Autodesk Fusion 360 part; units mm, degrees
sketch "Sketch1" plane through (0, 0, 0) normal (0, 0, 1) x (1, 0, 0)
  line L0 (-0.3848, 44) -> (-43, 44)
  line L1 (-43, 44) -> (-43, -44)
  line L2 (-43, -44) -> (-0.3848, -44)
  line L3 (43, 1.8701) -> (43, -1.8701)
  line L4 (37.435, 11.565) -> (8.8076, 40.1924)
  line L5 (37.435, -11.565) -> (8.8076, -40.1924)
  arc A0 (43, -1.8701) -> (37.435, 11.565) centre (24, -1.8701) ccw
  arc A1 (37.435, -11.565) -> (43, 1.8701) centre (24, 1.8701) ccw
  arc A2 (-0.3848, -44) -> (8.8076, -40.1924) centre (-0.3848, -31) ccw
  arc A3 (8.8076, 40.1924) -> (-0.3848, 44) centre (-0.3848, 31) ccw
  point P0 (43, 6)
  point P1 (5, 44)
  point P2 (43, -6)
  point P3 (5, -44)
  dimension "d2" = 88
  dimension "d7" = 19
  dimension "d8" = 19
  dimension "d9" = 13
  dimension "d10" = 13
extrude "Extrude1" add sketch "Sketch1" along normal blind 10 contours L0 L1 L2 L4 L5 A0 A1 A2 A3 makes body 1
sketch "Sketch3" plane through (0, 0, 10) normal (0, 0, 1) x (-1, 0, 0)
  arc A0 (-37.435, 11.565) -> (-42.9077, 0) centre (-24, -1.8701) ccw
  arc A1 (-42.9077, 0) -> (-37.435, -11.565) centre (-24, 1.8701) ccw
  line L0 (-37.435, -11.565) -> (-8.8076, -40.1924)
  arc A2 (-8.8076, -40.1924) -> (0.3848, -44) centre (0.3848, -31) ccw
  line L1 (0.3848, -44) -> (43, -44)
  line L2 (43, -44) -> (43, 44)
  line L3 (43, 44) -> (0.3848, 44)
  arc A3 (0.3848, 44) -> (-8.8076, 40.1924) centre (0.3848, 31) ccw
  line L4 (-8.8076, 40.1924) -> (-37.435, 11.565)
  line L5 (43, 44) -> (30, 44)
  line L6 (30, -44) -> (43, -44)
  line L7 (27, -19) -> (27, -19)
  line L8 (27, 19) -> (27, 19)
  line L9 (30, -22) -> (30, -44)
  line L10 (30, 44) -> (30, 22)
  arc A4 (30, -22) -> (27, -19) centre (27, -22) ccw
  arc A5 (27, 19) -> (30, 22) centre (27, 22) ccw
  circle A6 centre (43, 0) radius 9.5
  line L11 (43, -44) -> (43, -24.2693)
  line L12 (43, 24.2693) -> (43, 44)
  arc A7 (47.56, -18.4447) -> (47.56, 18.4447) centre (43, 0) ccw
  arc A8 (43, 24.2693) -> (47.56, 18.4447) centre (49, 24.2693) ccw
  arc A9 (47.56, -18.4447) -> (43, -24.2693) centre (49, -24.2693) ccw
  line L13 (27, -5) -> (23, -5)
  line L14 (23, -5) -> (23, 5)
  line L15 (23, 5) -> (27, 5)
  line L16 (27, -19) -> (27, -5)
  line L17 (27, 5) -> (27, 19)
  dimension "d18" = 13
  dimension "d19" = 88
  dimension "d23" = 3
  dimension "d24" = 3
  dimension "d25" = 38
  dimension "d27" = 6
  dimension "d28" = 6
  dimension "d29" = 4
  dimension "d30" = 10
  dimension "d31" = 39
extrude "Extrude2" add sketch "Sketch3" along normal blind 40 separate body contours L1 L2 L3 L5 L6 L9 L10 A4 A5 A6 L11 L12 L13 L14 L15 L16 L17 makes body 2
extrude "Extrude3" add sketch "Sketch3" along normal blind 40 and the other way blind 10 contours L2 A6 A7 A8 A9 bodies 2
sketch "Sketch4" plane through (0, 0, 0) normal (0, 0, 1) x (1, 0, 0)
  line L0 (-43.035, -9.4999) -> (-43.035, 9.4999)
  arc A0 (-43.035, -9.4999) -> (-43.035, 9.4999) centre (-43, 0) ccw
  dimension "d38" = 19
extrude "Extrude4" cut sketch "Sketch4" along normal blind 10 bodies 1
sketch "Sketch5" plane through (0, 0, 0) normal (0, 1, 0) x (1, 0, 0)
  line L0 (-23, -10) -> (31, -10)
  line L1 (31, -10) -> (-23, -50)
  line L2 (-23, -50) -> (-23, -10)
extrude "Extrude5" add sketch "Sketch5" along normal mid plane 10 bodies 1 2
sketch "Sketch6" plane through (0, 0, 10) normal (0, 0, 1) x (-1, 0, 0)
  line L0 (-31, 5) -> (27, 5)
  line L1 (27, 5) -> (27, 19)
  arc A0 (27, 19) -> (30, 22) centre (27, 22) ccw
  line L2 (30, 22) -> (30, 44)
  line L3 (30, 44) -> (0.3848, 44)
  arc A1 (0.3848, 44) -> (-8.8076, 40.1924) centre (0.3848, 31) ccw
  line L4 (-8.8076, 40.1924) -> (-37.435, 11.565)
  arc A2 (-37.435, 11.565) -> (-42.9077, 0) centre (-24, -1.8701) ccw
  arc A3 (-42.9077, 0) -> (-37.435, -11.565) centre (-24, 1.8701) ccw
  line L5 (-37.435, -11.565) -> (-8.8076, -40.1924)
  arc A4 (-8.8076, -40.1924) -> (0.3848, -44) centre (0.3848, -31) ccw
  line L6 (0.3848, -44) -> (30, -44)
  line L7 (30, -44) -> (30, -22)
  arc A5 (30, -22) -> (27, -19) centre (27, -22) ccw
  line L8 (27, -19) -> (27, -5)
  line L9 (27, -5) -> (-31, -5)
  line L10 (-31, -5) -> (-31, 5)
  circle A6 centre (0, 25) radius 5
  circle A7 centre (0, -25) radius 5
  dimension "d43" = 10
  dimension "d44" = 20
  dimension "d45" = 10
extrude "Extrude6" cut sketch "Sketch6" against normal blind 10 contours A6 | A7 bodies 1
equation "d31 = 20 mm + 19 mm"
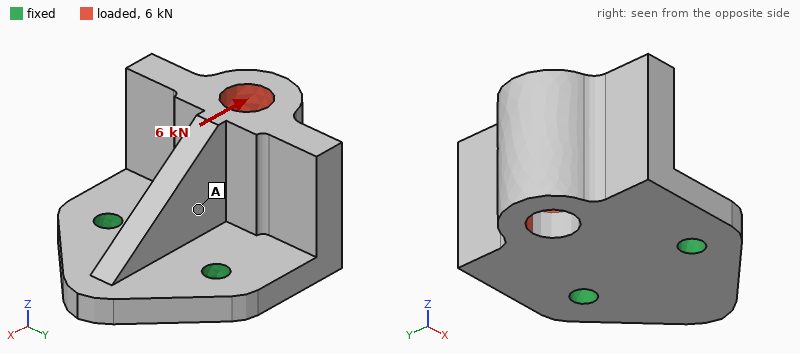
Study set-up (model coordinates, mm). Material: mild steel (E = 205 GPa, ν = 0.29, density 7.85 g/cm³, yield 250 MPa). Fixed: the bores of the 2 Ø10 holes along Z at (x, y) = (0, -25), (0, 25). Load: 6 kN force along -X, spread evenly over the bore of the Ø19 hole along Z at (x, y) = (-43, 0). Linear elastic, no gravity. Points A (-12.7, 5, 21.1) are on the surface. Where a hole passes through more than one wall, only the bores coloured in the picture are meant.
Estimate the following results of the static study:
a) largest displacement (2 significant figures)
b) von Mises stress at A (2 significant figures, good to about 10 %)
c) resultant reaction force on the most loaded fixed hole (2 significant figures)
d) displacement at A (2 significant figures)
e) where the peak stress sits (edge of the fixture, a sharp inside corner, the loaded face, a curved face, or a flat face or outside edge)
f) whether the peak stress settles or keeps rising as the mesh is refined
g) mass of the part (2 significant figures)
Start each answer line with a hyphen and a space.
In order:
- 63 µm
- 17 MPa
- 3.0 kN
- 15 µm
- edge of the fixture
- keeps rising
- 1.1 kg
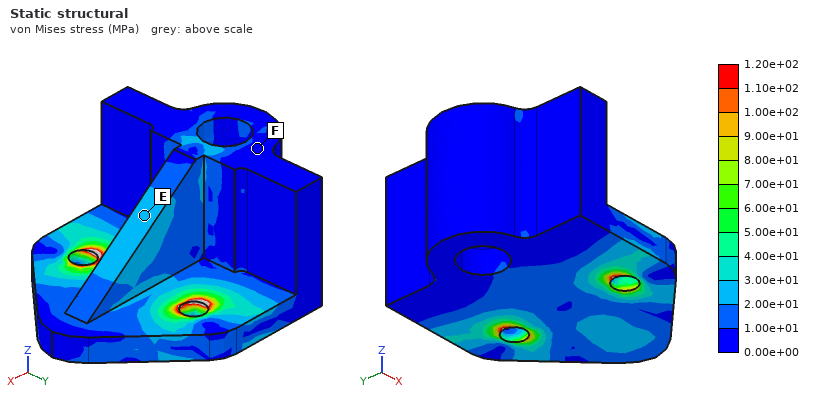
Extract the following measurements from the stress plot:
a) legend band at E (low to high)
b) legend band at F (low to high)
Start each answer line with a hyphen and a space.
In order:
- 2.00e+01 to 3.00e+01 MPa
- 0.00e+00 to 1.00e+01 MPa
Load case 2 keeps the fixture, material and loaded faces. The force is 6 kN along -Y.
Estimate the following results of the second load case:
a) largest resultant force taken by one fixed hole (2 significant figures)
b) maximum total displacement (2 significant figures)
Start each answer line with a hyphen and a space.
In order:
- 6.0 kN
- 30 µm
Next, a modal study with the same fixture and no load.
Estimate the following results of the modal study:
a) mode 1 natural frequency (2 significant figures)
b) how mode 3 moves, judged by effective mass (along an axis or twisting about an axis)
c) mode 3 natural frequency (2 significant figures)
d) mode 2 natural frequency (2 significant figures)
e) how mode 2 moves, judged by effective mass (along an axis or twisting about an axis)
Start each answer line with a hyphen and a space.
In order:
- 1700 Hz
- along Y
- 6500 Hz
- 3100 Hz
- along Y
